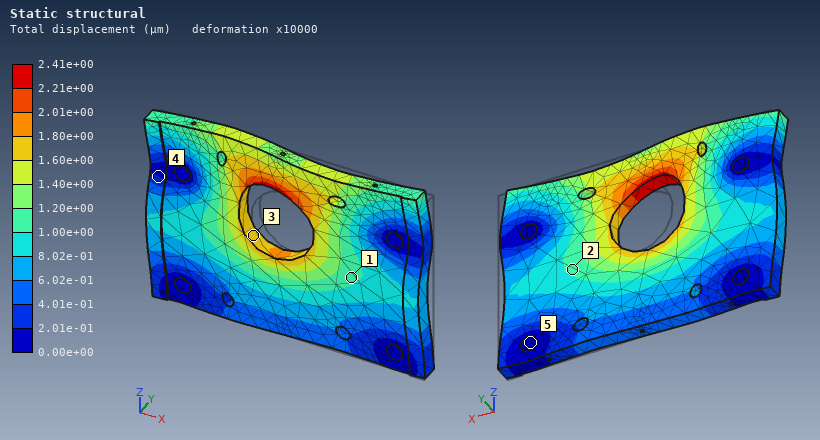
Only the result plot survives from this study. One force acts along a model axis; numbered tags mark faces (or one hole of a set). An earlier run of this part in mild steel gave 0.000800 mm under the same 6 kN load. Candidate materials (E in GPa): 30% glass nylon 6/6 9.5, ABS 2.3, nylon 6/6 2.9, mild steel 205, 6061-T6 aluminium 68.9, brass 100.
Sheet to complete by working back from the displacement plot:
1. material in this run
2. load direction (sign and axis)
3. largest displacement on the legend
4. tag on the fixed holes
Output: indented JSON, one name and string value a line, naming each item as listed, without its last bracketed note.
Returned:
{
  "material in this run": "6061-T6 aluminium",
  "load direction": "-X",
  "largest displacement on the legend": "2.41e+00 µm",
  "tag on the fixed holes": "5"
}
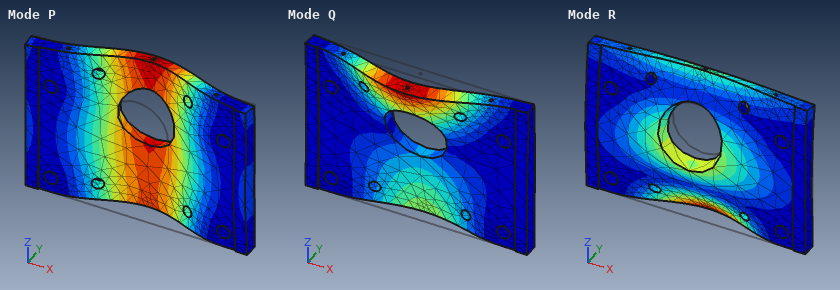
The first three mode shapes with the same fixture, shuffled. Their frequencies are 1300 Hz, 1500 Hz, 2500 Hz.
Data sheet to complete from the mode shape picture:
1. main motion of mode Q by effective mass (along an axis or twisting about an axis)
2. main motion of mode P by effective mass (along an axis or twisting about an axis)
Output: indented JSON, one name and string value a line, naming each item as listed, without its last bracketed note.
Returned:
{
  "main motion of mode Q by effective mass": "twisting about X",
  "main motion of mode P by effective mass": "along Y"
}
